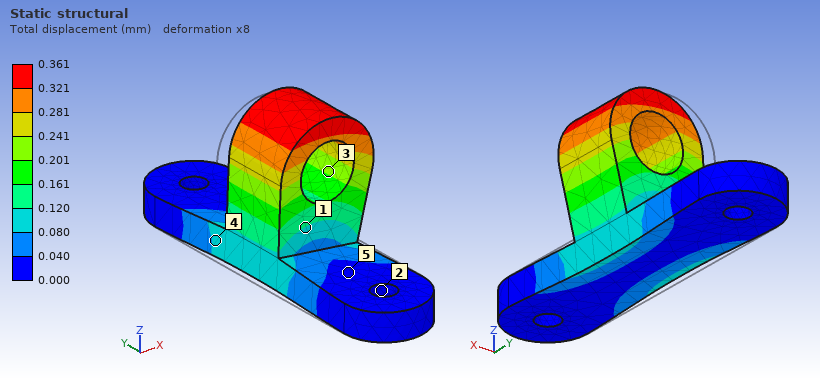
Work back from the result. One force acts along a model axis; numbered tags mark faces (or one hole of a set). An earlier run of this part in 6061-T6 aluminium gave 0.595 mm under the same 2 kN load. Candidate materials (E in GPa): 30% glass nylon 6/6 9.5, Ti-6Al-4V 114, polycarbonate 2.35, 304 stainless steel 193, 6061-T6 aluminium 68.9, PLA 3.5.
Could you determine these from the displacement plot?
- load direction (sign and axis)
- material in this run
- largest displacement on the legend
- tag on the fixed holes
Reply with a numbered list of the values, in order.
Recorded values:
1. +X
2. Ti-6Al-4V
3. 0.361 mm
4. 2
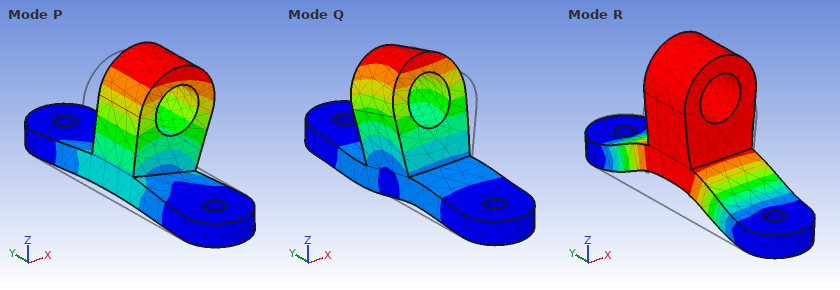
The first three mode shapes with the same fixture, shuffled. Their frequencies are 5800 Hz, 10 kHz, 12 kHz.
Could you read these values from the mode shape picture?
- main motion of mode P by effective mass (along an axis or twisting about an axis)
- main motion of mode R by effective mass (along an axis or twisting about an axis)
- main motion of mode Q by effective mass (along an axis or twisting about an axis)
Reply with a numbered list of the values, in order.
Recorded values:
1. along X
2. along Z
3. along Y
